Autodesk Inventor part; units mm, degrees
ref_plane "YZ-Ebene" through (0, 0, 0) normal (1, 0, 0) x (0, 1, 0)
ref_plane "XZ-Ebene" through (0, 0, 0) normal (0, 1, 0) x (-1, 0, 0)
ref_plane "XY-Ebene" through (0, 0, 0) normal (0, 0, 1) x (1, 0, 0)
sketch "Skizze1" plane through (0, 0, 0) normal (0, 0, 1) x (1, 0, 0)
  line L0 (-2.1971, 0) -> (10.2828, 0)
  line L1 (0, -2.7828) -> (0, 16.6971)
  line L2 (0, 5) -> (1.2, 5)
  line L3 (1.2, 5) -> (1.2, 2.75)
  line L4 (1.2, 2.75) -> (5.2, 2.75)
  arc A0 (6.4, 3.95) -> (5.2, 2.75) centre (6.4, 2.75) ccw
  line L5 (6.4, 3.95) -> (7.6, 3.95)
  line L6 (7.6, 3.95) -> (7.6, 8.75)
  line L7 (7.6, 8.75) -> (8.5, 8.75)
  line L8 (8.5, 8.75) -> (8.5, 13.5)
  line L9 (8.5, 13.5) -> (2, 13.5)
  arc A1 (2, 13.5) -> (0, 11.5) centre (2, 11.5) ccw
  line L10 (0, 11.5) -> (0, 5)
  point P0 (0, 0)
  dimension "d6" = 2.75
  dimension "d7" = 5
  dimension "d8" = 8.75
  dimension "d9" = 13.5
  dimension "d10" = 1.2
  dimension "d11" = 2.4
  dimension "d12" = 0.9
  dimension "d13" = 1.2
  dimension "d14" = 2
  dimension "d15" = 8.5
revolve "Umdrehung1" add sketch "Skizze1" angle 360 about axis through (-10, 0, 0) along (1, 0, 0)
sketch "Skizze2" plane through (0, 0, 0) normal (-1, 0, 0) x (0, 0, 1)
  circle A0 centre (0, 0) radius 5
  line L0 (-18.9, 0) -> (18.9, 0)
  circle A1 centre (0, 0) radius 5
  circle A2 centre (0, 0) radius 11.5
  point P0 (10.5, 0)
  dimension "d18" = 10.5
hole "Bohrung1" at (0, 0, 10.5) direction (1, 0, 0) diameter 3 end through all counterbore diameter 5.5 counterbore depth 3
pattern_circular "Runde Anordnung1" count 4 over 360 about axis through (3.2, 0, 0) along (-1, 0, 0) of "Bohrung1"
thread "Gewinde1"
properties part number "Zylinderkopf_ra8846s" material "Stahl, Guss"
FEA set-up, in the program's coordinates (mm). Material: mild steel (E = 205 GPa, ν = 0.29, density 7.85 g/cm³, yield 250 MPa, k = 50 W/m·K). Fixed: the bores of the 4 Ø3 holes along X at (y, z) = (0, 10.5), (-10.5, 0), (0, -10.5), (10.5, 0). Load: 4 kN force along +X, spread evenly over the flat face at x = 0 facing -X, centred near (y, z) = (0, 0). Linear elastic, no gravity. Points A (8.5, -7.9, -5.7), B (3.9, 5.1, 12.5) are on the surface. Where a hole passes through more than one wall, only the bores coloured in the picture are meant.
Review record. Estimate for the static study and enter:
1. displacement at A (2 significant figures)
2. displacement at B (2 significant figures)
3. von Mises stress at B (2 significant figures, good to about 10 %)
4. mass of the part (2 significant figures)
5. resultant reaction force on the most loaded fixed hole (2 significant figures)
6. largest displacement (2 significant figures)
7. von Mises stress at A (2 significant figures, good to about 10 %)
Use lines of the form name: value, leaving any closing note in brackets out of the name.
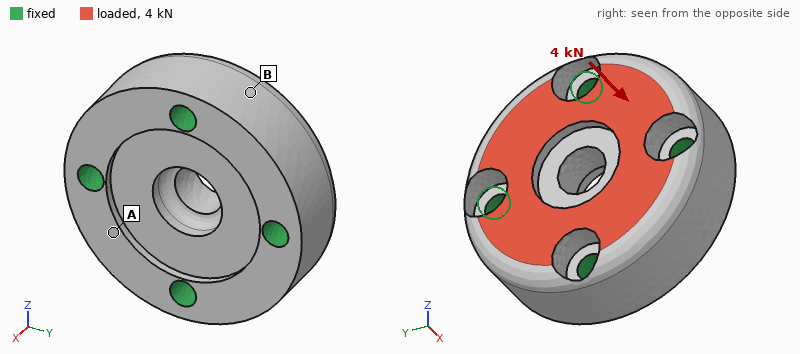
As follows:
displacement at A: 0.74 µm
displacement at B: 0.51 µm
von Mises stress at B: 7.4 MPa
mass of the part: 30 g
resultant reaction force on the most loaded fixed hole: 1.0 kN
largest displacement: 1.2 µm
von Mises stress at A: 13 MPa
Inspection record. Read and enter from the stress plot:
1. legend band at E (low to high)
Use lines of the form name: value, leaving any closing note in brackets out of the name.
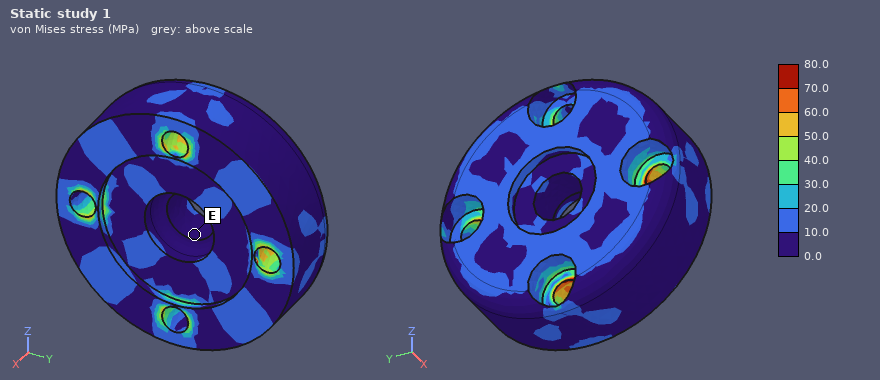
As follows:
legend band at E: 0.0 to 10.0 MPa
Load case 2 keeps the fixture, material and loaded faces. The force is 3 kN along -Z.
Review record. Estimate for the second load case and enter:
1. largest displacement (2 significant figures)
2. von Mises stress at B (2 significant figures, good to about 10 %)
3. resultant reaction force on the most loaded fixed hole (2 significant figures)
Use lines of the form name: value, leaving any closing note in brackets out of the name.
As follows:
largest displacement: 1.5 µm
von Mises stress at B: 15 MPa
resultant reaction force on the most loaded fixed hole: 1.0 kN
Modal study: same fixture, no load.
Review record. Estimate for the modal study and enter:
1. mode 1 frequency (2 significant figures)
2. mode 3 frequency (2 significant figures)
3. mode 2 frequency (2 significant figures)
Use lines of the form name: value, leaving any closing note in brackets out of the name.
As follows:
mode 1 frequency: 63 kHz
mode 3 frequency: 65 kHz
mode 2 frequency: 65 kHz
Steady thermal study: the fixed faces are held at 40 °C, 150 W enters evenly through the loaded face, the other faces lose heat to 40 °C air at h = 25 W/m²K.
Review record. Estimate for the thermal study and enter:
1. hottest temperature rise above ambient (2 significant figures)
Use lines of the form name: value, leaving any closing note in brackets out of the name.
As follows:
hottest temperature rise above ambient: 75 K
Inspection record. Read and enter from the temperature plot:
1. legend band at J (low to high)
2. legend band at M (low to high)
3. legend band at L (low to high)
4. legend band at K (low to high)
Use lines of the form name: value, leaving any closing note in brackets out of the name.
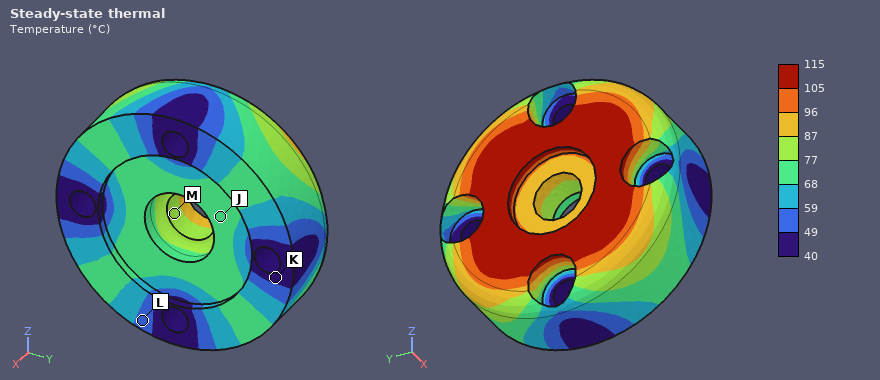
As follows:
legend band at J: 68 to 77 °C
legend band at M: 77 to 87 °C
legend band at L: 49 to 59 °C
legend band at K: 40 to 49 °C
